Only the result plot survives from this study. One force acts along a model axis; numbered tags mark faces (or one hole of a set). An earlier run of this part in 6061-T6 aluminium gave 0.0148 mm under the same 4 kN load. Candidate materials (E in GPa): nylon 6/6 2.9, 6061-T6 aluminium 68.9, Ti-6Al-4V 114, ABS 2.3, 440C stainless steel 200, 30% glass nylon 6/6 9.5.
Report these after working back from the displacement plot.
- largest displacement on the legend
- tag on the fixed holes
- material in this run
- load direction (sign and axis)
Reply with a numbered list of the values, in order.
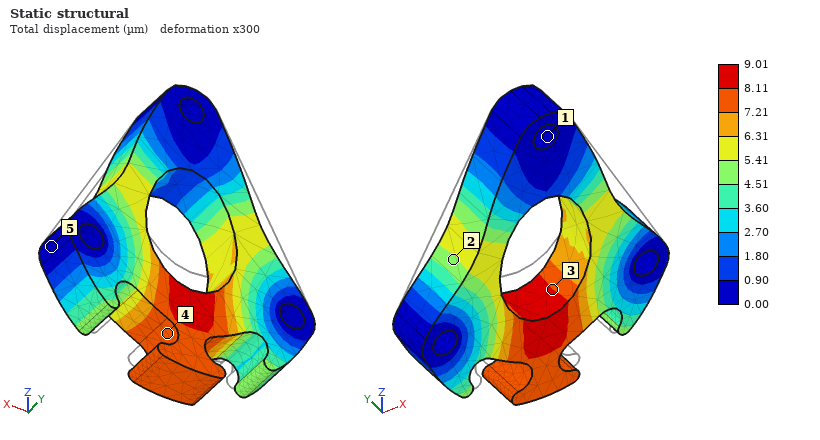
1. 9.01 µm
2. 1
3. Ti-6Al-4V
4. -Z
